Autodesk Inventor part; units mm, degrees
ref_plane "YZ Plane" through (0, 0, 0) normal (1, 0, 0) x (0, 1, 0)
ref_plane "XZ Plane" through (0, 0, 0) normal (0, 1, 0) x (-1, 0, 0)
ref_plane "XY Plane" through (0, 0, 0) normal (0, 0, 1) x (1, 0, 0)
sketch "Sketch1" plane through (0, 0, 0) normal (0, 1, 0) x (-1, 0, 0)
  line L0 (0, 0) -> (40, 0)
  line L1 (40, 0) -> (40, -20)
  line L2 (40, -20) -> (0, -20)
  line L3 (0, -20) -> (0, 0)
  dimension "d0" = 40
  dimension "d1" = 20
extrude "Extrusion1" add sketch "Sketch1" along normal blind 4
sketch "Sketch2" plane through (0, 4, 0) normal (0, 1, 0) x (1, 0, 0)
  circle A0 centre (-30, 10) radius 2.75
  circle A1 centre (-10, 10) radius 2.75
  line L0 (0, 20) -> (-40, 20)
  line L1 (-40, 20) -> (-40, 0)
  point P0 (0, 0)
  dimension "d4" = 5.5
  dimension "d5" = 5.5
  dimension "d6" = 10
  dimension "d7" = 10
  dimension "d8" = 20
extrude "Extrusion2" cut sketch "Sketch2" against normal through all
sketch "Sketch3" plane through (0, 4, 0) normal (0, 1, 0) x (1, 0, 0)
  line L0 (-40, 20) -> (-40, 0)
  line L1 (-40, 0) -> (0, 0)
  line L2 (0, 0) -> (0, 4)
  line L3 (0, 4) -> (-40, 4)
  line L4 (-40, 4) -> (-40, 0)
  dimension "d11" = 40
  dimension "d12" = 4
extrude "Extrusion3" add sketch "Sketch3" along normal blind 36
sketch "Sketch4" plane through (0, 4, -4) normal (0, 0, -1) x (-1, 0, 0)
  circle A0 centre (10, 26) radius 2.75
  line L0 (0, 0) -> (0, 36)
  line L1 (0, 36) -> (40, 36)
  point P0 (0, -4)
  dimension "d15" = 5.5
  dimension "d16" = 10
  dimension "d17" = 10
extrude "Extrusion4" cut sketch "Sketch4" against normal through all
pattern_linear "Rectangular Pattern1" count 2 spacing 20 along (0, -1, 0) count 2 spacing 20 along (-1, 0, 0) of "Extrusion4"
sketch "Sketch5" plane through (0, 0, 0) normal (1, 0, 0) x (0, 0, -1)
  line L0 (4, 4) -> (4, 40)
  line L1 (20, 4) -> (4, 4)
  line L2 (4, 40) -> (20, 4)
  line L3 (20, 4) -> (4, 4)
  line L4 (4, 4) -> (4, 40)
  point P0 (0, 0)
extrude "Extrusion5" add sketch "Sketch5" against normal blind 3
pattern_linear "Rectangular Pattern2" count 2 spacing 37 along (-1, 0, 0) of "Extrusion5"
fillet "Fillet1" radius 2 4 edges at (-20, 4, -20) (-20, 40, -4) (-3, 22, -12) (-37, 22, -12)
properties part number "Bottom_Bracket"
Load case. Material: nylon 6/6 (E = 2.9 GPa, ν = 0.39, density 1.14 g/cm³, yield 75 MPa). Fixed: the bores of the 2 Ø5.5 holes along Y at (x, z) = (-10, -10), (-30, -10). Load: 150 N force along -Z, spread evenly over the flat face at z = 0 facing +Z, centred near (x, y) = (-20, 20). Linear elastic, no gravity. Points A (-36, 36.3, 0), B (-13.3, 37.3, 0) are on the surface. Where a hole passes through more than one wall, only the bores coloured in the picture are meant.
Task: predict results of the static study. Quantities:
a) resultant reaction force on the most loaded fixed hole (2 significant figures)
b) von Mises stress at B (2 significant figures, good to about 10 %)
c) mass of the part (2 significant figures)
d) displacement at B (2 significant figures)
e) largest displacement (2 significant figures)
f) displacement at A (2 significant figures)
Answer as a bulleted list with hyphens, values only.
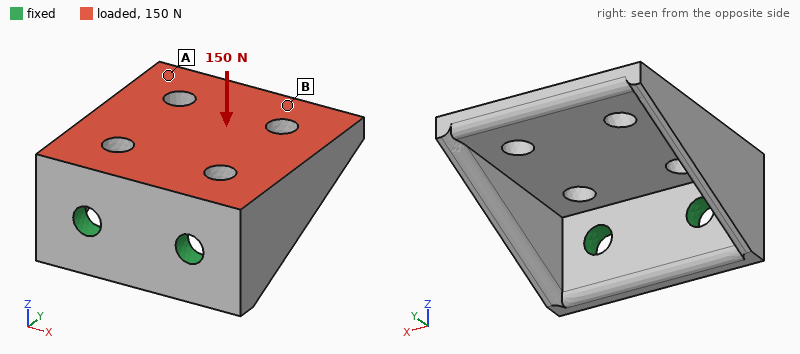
- 75 N
- 4.8 MPa
- 11 g
- 0.61 mm
- 0.68 mm
- 0.52 mm
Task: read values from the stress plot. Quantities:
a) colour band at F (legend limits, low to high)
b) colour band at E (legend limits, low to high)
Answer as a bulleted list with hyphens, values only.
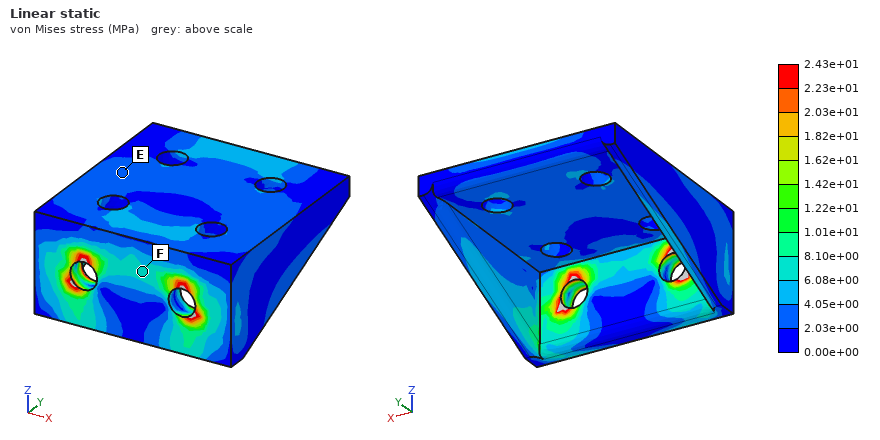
- 6.08e+00 to 8.10e+00 MPa
- 2.03e+00 to 4.05e+00 MPa
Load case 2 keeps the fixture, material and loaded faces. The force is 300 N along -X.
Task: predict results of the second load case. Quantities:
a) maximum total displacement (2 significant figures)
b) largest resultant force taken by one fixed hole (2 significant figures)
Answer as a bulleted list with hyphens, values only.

- 0.33 mm
- 270 N
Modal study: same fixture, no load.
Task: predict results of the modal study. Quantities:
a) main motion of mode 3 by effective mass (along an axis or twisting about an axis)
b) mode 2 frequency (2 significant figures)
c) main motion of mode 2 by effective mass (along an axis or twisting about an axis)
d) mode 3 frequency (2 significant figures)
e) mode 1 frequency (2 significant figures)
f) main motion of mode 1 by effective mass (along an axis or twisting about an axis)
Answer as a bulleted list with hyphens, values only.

- along X
- 1600 Hz
- along X
- 2900 Hz
- 1100 Hz
- along Z
